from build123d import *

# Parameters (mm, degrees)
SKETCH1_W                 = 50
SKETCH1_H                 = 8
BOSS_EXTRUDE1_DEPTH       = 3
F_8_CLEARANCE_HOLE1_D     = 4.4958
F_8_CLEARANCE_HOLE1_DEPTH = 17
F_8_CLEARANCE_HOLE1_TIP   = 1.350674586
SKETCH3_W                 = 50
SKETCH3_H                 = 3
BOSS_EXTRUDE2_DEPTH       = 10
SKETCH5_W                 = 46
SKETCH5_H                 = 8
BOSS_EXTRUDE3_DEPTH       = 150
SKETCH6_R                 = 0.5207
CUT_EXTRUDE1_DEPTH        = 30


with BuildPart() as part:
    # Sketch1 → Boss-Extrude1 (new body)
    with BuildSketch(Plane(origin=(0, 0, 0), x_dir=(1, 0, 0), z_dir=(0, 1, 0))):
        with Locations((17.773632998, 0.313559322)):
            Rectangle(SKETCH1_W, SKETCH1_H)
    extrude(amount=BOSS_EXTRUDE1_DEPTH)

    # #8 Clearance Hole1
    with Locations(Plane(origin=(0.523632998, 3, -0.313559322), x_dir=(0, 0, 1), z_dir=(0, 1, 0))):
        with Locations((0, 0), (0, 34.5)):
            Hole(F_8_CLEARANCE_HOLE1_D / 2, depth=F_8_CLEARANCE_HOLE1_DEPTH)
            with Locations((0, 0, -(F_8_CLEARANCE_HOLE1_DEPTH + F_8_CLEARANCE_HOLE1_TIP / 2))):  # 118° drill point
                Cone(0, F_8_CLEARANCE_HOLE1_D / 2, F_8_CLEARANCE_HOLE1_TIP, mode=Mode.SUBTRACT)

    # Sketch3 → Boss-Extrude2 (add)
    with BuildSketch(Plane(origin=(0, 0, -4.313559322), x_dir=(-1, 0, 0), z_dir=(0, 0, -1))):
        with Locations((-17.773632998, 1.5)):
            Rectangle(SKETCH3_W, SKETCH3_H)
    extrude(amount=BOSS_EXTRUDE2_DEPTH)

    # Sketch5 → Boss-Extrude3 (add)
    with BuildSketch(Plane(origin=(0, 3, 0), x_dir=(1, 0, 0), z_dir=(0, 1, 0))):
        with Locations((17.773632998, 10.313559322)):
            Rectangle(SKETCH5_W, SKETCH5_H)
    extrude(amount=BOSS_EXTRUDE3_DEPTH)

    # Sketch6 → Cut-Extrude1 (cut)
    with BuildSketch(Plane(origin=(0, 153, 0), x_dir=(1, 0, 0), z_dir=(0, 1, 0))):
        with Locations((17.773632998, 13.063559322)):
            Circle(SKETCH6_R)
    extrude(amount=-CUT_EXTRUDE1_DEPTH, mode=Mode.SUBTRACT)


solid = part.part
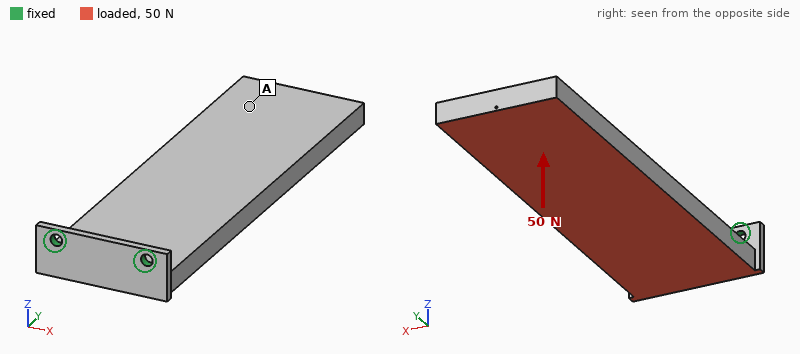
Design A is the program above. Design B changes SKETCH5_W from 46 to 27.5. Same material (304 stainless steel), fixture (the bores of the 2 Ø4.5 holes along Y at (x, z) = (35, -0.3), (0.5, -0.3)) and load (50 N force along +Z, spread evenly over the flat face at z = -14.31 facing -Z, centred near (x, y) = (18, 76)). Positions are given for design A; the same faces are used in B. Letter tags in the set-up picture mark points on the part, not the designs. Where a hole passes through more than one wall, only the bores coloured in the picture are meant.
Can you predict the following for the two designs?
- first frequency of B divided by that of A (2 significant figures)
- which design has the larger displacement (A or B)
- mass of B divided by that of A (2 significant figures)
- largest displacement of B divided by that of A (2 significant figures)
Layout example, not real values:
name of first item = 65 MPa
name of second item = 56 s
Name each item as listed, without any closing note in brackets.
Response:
first frequency of B divided by that of A = 1.1
which design has the larger displacement = B
mass of B divided by that of A = 0.62
largest displacement of B divided by that of A = 1.3
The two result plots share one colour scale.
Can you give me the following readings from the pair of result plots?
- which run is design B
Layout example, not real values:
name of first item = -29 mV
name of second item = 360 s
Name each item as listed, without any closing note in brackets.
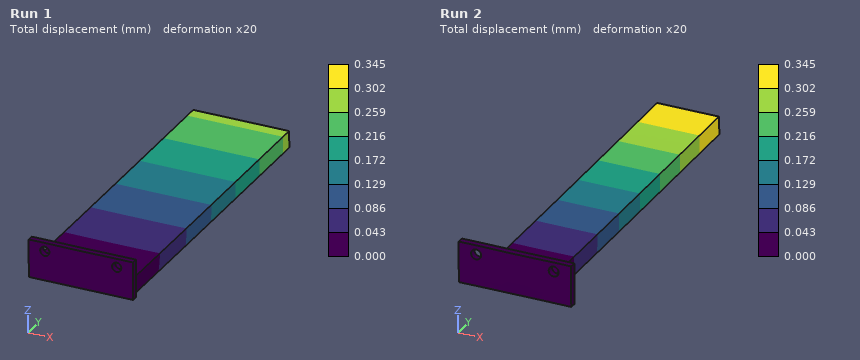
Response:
which run is design B = Run 2
